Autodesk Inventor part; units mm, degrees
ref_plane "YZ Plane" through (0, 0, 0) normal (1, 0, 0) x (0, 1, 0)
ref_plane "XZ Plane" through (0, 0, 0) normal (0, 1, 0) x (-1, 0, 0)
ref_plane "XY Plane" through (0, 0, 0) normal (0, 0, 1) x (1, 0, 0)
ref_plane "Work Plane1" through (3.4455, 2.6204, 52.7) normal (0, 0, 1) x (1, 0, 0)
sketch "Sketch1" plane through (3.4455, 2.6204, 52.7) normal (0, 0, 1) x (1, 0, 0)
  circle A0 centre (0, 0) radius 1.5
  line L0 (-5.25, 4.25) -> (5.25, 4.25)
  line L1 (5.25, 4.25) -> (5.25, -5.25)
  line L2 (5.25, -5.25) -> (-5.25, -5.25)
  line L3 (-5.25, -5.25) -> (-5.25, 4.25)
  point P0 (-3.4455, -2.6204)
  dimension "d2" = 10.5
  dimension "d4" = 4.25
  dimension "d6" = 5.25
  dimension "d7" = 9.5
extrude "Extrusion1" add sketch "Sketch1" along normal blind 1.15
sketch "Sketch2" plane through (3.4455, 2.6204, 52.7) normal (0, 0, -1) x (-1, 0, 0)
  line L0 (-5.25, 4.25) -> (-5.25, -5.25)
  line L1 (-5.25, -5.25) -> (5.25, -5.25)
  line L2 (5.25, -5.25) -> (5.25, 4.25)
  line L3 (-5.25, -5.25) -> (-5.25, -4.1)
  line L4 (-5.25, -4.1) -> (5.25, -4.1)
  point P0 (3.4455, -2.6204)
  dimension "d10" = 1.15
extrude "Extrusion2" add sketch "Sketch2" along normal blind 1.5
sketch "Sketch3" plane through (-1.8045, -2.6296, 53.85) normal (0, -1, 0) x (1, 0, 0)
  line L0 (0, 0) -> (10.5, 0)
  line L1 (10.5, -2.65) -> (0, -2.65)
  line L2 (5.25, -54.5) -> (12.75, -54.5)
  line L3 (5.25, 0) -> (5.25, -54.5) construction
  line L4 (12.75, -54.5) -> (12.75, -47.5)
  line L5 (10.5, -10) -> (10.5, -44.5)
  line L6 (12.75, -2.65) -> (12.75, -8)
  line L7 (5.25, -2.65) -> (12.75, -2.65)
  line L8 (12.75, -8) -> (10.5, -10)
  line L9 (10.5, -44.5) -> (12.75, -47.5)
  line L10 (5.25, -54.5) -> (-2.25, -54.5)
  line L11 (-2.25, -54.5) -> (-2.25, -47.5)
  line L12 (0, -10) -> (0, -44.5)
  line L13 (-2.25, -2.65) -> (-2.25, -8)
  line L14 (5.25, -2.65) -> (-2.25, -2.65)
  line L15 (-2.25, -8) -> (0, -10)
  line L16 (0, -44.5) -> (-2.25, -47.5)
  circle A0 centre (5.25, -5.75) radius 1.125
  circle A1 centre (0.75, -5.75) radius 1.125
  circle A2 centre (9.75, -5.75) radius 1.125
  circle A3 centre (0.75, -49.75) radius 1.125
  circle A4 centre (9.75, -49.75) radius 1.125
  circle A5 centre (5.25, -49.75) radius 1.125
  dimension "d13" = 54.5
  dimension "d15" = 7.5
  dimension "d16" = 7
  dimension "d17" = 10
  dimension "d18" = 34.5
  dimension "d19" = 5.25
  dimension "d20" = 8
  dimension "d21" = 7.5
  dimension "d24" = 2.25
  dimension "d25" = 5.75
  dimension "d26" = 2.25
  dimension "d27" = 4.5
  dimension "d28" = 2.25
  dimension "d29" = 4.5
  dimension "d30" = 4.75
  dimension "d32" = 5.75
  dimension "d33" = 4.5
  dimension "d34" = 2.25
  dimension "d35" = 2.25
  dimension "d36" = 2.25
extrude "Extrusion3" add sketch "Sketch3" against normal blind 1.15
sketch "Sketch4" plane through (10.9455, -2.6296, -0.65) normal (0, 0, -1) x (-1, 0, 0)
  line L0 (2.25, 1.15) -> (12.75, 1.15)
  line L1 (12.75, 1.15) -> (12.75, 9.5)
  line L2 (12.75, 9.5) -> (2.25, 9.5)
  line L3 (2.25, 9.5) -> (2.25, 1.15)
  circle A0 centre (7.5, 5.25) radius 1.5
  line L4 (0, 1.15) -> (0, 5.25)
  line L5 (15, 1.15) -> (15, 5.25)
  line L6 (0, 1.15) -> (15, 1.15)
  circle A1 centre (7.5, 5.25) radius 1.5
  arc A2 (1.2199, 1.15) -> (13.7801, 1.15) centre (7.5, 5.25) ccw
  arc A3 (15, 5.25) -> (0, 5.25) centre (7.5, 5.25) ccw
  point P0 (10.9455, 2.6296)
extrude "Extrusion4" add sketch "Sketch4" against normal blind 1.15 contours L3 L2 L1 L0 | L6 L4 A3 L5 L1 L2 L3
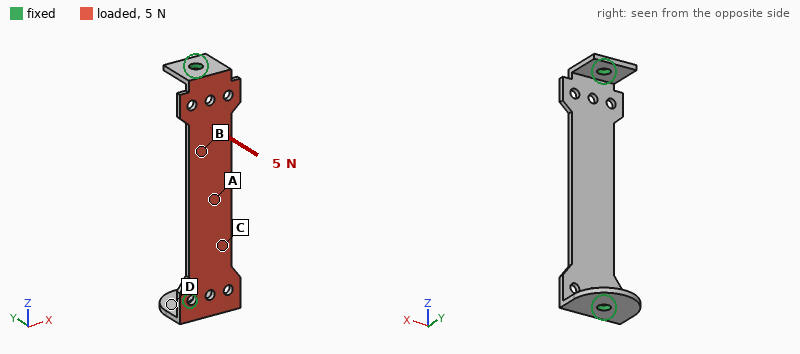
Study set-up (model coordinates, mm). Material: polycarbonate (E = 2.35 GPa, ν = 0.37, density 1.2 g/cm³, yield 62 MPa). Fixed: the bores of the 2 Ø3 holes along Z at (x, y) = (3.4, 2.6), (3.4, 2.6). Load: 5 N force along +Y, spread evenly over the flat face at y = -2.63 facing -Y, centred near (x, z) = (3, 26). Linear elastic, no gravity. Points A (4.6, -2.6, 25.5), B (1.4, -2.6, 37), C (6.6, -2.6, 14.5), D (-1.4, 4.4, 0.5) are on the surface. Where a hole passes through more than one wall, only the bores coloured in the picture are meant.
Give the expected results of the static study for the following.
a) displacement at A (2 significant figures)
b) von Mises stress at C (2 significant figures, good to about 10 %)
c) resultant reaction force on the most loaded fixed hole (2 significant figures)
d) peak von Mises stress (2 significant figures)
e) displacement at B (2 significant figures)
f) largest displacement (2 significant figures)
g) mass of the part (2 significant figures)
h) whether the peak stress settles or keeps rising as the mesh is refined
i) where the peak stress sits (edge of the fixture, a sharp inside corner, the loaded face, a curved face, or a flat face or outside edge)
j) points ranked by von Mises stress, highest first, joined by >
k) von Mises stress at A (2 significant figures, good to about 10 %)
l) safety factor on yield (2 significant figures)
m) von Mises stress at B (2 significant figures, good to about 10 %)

0.63 mm
2.3 MPa
6.3 N
12 MPa
0.47 mm
0.65 mm
1.2 g
settles
a curved face
A > B > C > D
4.9 MPa
5.4
3.1 MPa
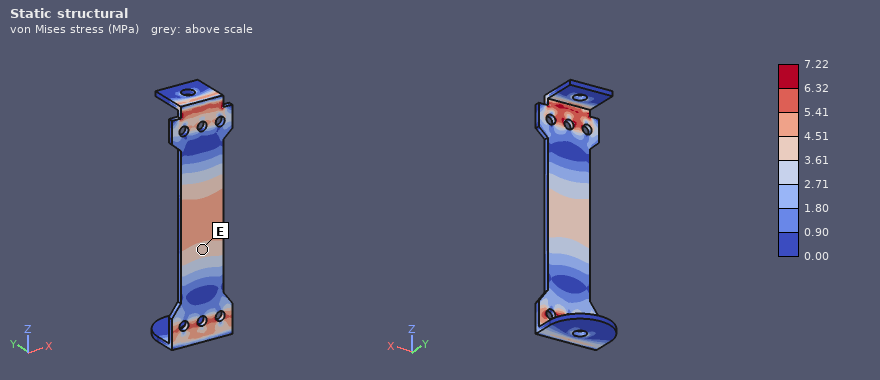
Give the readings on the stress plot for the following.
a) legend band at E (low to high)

3.61 to 4.51 MPa
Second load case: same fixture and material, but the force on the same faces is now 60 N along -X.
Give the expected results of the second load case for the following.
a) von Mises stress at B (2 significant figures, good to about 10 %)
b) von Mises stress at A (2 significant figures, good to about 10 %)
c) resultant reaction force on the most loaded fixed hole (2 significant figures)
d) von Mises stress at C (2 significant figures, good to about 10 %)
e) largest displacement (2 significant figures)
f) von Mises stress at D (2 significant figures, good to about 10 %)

6.1 MPa
3.2 MPa
31 N
7.9 MPa
0.49 mm
3.9 MPa
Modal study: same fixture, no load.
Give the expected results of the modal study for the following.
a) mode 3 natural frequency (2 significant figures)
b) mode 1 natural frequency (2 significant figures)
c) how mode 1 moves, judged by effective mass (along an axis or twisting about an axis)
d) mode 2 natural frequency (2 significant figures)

1800 Hz
560 Hz
along Y
1400 Hz
